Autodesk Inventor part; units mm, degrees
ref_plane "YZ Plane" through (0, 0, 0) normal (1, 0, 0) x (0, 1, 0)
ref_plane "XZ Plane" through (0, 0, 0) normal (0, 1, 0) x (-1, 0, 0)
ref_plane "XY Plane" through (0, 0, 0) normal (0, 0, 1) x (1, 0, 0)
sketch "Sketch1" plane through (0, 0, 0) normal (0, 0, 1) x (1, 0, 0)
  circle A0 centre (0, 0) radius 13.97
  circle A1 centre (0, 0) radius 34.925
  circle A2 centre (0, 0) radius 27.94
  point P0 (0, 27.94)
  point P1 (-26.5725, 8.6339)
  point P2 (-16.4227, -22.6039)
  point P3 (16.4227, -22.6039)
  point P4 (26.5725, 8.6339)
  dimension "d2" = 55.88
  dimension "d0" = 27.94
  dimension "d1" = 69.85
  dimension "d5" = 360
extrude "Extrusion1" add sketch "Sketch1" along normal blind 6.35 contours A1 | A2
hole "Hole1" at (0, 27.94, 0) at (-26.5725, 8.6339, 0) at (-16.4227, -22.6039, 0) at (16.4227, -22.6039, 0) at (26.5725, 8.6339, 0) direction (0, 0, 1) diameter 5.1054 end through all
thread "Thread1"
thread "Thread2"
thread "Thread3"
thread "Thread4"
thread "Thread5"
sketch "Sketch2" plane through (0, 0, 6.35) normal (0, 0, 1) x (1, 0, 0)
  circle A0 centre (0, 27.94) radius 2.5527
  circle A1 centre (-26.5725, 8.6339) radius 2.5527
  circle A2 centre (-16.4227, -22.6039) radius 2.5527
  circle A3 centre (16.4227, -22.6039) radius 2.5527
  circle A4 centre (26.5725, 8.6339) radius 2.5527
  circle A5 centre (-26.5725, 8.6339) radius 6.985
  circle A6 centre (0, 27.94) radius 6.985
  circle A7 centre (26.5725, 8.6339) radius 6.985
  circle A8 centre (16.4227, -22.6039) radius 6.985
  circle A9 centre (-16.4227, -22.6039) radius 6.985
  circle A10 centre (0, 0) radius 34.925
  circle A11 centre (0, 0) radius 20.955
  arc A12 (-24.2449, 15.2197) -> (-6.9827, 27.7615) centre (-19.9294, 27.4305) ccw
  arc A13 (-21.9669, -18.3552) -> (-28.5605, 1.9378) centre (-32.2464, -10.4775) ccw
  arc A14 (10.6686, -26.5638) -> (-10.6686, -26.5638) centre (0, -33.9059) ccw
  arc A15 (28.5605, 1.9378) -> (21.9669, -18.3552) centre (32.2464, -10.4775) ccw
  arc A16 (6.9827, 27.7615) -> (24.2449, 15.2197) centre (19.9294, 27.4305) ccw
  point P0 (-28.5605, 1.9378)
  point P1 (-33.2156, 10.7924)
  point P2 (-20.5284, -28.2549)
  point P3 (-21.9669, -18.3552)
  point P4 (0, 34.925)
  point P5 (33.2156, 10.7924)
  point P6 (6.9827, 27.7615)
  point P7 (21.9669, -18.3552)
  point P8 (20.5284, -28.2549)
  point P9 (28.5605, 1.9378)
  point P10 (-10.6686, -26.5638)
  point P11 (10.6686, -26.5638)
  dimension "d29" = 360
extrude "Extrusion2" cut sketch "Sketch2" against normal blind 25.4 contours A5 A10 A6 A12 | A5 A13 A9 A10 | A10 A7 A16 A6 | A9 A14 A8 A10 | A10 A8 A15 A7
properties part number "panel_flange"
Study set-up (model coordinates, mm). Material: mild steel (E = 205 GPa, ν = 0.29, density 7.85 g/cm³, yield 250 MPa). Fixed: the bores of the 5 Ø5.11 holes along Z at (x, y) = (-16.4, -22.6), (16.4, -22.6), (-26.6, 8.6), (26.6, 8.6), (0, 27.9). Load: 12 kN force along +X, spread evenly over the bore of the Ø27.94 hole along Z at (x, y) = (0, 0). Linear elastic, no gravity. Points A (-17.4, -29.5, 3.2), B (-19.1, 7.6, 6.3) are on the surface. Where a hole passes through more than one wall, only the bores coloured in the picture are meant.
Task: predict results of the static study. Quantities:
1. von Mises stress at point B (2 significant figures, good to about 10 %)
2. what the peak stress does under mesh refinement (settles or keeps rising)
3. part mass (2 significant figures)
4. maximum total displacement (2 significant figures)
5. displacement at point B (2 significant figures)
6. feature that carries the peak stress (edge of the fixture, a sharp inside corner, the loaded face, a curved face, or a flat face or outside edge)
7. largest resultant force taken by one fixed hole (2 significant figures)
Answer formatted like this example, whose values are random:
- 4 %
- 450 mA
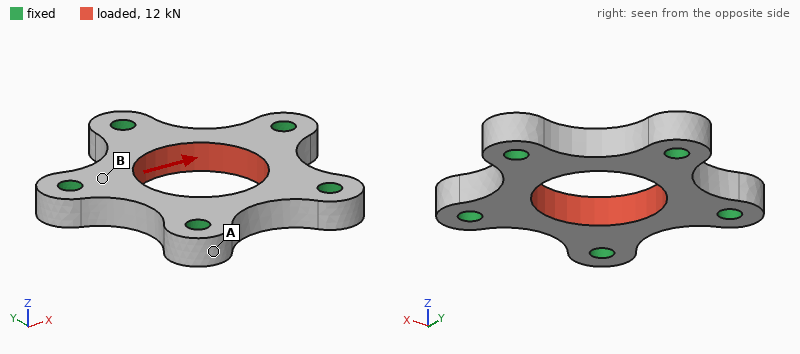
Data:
- 36 MPa
- keeps rising
- 82 g
- 4.4 µm
- 1.1 µm
- edge of the fixture
- 3.5 kN
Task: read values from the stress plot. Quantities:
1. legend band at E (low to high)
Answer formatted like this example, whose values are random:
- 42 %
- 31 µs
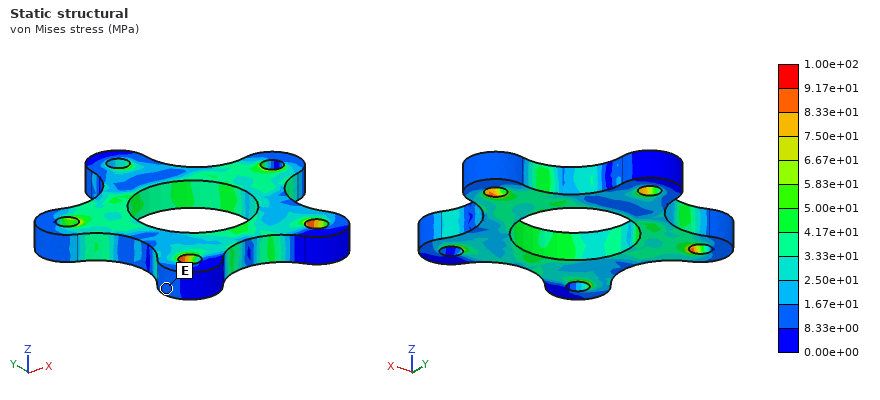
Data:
- 8.33e+00 to 1.67e+01 MPa
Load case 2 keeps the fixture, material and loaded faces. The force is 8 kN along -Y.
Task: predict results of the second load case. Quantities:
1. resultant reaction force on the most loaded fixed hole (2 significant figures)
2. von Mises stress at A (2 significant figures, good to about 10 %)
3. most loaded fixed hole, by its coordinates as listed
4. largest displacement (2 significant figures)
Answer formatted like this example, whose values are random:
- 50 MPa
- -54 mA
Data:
- 2.5 kN
- 7.4 MPa
- (0, 27.9)
- 2.9 µm
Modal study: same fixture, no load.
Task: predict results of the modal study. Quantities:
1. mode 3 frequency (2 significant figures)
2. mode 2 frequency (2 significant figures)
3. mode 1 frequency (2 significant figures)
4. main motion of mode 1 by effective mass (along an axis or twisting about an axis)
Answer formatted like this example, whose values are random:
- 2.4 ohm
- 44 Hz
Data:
- 27 kHz
- 27 kHz
- 23 kHz
- along Z
